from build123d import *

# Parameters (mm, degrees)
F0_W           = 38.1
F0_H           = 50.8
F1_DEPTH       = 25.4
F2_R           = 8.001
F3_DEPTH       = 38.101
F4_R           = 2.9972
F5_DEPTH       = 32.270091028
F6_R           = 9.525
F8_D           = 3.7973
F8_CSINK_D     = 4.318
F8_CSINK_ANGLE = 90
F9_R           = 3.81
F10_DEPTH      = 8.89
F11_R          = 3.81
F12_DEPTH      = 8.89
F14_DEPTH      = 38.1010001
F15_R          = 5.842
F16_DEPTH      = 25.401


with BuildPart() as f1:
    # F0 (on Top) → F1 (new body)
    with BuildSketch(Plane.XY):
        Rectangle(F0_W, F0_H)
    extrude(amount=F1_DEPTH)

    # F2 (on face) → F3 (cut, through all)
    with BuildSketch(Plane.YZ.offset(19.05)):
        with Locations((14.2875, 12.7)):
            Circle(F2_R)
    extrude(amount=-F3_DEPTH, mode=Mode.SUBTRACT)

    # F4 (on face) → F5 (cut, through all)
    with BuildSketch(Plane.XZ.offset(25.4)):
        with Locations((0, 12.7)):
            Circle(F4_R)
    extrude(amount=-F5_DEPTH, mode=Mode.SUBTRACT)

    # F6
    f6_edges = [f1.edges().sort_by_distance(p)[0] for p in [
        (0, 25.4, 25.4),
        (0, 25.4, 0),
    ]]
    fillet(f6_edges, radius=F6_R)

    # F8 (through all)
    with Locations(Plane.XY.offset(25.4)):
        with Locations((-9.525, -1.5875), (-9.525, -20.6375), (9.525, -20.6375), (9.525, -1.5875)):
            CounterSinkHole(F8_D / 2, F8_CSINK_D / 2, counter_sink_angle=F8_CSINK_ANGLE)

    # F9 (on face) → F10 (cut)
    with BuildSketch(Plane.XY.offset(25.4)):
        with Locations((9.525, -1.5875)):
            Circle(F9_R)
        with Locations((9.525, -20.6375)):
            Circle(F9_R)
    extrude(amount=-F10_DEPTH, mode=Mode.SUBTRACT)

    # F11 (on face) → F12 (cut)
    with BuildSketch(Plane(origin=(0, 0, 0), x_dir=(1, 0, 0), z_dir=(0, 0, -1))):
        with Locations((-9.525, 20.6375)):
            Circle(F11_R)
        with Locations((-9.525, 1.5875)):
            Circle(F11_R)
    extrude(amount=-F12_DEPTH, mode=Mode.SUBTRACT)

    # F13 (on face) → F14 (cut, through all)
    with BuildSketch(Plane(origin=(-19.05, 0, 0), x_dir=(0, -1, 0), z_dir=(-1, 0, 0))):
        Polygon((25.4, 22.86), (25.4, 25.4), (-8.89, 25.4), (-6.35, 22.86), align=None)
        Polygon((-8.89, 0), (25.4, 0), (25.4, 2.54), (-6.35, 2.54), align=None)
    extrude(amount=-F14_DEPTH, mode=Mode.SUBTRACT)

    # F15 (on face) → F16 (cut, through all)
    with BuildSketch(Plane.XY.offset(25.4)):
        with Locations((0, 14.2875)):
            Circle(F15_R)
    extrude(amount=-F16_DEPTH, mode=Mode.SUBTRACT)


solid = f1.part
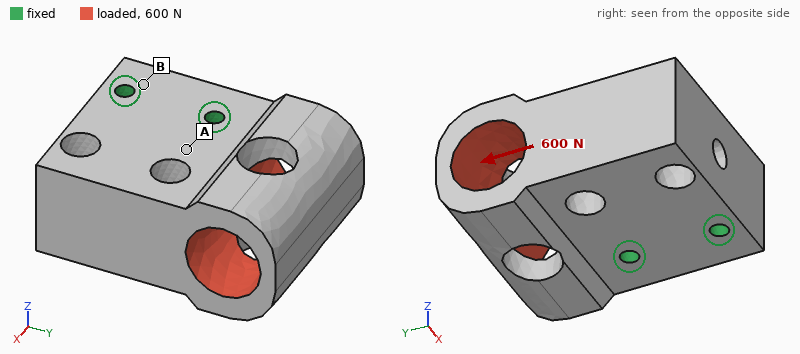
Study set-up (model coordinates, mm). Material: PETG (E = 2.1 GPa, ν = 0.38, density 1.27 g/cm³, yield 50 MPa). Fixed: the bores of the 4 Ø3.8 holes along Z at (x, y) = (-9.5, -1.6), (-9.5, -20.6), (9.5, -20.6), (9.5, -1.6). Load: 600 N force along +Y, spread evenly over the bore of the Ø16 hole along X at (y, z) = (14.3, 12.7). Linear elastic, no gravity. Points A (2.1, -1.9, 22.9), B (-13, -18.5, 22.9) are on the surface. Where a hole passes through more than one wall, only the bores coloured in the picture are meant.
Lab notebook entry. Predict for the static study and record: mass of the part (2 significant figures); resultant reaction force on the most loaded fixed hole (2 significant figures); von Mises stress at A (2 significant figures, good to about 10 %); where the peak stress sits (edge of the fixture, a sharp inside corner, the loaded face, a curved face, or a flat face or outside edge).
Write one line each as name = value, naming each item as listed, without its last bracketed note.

mass of the part = 38 g
resultant reaction force on the most loaded fixed hole = 230 N
von Mises stress at A = 1.0 MPa
where the peak stress sits = the loaded face
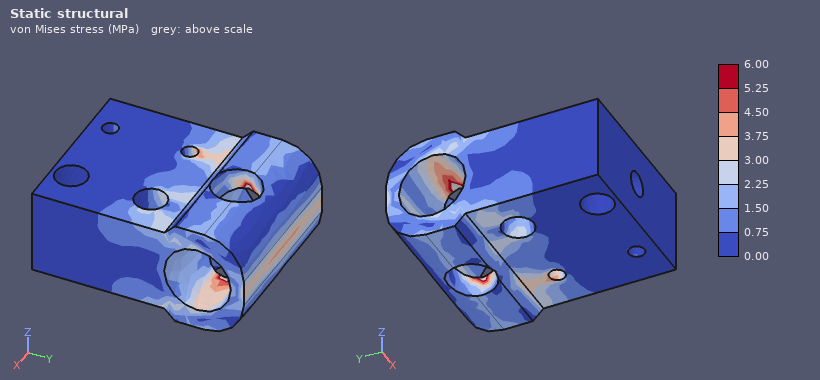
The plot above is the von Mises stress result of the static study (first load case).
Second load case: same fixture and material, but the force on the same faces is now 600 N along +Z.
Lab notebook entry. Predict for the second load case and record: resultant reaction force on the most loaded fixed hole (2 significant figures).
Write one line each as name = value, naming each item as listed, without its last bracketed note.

resultant reaction force on the most loaded fixed hole = 400 N
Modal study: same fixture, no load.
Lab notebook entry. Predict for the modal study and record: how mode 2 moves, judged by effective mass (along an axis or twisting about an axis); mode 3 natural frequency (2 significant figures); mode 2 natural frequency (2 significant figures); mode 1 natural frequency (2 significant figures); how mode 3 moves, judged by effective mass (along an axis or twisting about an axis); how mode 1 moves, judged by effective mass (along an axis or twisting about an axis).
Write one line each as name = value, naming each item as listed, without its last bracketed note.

how mode 2 moves, judged by effective mass = along X
mode 3 natural frequency = 4500 Hz
mode 2 natural frequency = 3800 Hz
mode 1 natural frequency = 2500 Hz
how mode 3 moves, judged by effective mass = twisting about Y
how mode 1 moves, judged by effective mass = along Z
